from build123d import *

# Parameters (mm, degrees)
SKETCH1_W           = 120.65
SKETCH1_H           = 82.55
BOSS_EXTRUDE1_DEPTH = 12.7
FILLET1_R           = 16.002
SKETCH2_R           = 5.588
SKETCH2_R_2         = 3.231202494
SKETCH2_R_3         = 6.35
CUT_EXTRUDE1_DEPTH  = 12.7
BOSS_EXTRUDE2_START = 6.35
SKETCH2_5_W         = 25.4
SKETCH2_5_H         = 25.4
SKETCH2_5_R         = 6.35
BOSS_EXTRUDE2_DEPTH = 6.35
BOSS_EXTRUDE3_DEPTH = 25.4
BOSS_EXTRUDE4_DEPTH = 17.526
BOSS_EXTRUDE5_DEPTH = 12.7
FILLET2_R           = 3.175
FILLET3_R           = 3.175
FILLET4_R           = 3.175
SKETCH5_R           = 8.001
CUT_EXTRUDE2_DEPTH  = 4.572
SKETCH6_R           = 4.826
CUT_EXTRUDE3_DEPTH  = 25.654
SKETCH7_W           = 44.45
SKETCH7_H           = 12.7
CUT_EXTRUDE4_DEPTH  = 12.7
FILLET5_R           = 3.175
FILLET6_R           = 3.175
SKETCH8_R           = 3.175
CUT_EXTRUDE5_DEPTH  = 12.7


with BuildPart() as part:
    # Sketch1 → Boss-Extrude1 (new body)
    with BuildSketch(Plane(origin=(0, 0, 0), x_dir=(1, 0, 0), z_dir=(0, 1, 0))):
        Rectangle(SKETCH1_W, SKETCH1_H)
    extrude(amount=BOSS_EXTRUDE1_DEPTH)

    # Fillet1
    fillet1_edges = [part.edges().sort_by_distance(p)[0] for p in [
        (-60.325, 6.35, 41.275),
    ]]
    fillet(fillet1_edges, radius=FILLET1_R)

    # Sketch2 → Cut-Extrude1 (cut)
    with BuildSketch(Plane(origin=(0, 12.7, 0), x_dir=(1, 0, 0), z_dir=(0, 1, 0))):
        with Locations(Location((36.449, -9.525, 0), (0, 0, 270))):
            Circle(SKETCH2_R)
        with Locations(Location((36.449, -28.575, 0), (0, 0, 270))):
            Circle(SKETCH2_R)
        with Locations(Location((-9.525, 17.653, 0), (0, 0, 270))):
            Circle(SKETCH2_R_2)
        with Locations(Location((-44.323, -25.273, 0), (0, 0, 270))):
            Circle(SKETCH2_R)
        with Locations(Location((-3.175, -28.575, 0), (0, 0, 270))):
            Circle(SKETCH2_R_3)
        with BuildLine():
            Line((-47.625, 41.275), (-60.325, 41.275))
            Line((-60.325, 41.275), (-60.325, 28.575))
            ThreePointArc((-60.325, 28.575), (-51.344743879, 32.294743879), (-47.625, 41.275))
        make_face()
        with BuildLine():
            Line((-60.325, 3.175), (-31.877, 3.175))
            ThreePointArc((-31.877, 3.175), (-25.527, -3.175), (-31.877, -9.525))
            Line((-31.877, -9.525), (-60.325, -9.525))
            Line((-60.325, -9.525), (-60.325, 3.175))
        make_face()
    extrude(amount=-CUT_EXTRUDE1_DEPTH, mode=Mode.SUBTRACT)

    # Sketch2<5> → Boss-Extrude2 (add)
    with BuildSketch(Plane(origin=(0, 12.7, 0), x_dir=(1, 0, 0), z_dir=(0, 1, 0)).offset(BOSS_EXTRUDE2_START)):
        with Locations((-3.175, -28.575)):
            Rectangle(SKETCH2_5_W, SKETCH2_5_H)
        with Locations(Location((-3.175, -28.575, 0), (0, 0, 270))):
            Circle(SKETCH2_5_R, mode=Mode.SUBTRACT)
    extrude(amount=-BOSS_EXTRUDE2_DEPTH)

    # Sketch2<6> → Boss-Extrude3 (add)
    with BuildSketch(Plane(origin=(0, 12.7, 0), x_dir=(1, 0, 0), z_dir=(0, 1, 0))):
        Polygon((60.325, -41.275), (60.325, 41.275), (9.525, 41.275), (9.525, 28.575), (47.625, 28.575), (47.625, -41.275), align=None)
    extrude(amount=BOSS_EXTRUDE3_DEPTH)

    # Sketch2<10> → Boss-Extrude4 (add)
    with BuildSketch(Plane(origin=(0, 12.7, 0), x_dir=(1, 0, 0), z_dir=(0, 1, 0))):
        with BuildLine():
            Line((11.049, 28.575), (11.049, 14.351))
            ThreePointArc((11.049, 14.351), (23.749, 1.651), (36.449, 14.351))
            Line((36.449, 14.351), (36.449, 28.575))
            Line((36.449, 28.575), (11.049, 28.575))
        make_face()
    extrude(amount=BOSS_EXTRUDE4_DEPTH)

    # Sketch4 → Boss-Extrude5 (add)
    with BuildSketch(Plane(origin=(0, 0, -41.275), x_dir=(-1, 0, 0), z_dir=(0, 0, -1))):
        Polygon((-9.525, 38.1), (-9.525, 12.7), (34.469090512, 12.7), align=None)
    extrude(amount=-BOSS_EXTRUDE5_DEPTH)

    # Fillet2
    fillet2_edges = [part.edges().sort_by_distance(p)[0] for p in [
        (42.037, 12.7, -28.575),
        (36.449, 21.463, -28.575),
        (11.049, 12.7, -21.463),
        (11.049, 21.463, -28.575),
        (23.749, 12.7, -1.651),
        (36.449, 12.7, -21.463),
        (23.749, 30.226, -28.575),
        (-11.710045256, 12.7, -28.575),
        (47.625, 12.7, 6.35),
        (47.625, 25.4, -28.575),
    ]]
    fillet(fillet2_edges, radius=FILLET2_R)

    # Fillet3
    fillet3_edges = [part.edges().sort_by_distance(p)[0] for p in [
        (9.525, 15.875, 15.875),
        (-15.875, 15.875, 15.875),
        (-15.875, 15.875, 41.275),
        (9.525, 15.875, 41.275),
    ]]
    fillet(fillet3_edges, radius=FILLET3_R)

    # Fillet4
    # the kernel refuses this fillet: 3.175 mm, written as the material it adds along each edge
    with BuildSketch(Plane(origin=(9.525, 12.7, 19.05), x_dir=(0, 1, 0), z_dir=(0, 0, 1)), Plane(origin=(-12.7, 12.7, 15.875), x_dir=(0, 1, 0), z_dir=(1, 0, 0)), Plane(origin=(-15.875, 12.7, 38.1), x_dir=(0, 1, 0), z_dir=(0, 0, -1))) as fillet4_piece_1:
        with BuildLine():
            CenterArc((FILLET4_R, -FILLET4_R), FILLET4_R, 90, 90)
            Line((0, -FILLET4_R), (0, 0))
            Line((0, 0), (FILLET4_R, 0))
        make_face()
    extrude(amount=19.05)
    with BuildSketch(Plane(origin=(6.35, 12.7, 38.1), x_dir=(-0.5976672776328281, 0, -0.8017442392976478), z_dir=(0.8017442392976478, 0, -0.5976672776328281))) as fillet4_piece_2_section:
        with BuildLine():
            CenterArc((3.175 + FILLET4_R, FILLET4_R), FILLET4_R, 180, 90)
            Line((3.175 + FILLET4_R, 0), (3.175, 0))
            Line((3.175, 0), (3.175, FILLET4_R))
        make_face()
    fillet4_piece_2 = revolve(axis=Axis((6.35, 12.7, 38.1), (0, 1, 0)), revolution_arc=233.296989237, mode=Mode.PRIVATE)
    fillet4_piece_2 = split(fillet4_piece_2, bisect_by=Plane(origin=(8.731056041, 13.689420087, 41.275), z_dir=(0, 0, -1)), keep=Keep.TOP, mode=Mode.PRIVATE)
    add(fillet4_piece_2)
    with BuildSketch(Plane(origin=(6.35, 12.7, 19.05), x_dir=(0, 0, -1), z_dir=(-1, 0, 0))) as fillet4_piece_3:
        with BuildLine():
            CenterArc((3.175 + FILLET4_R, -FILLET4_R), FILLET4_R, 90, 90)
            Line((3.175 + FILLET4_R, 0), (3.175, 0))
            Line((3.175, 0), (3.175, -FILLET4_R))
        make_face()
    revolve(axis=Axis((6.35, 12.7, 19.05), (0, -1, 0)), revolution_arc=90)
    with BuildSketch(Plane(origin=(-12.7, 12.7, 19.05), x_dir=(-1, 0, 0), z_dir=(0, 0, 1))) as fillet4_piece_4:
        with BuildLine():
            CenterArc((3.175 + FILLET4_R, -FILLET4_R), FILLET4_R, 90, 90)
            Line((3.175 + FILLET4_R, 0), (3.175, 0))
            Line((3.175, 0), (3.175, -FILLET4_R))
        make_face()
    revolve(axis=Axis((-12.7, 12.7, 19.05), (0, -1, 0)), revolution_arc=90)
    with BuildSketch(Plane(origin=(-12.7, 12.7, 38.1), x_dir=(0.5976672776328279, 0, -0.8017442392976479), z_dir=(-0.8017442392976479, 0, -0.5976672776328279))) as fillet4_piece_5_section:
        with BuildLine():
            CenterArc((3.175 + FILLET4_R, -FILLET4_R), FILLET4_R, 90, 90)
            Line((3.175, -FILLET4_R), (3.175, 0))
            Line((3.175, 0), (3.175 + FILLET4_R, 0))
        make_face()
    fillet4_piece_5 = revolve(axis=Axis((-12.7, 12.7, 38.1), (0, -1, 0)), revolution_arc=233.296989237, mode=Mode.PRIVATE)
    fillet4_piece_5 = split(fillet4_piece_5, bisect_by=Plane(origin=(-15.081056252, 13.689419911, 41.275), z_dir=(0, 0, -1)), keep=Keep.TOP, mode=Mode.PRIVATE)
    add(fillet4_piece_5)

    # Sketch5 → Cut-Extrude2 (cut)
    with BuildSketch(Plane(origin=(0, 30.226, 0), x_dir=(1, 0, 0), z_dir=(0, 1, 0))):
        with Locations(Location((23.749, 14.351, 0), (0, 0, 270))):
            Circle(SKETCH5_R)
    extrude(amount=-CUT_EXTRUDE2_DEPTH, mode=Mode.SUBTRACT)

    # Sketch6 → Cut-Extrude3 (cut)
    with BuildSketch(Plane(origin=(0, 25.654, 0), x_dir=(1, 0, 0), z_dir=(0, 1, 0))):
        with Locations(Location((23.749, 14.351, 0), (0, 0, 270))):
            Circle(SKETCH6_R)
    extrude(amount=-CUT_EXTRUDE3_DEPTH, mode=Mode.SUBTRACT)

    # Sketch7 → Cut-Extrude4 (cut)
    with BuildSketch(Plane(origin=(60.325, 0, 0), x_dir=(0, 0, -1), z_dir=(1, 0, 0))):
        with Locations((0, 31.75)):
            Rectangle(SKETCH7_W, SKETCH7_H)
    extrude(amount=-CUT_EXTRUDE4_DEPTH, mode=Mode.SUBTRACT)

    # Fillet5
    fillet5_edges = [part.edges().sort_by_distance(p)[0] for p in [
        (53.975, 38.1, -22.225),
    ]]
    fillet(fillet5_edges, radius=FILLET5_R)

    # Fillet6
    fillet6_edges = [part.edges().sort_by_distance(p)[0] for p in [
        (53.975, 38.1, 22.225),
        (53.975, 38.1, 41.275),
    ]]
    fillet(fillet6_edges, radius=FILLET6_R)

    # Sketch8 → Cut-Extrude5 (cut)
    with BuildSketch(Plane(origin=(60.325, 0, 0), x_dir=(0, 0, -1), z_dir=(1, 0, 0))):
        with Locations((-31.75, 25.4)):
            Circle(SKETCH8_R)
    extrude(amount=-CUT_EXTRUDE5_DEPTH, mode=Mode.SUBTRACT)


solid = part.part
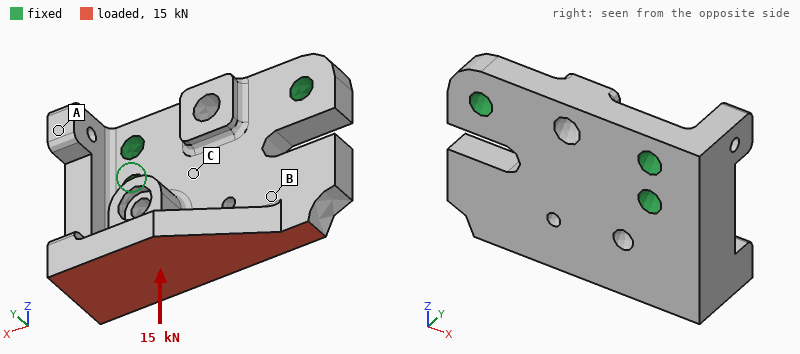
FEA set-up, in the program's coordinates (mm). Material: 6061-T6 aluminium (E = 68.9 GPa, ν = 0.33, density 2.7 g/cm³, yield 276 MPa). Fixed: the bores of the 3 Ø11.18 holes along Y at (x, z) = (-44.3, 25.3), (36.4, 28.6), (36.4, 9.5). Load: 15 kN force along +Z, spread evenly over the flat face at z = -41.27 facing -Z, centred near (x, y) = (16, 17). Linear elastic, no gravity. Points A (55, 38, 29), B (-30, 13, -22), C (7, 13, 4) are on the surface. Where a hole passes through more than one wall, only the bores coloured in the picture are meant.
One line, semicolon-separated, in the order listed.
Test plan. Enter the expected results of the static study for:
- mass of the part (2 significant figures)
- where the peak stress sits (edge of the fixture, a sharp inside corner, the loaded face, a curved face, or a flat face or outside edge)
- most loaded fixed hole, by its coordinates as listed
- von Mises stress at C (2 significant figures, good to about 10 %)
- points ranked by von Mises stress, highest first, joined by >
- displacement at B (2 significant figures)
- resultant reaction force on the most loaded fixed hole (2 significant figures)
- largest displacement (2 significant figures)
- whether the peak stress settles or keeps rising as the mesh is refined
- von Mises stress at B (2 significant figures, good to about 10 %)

440 g; edge of the fixture; (36.4, 9.5); 33 MPa; C > B > A; 0.079 mm; 7.9 kN; 0.15 mm; keeps rising; 18 MPa
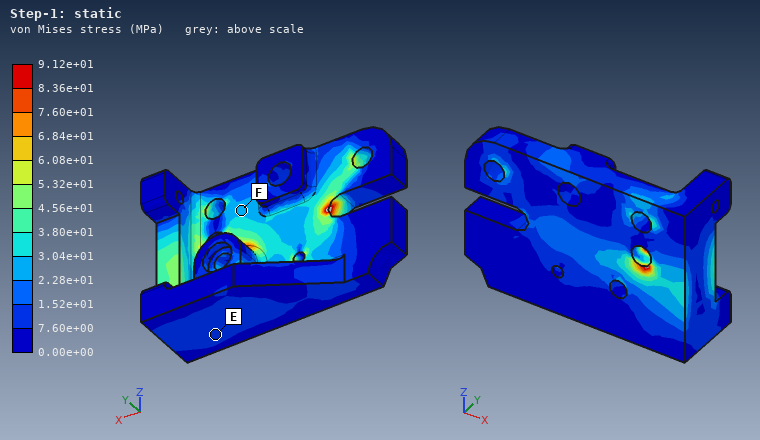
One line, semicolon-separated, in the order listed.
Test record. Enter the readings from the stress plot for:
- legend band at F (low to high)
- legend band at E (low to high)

2.28e+01 to 3.04e+01 MPa; 7.60e+00 to 1.52e+01 MPa
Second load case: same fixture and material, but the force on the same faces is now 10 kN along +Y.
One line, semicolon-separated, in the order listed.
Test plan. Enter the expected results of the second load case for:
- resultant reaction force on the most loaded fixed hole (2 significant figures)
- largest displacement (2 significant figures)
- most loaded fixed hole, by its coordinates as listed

18 kN; 0.55 mm; (36.4, 9.5)
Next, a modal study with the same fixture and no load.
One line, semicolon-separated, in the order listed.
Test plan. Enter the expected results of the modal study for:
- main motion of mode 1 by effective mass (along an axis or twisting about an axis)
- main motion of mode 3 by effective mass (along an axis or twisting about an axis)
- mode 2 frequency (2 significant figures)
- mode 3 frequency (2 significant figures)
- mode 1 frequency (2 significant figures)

along Y; along X; 3400 Hz; 5100 Hz; 2000 Hz
